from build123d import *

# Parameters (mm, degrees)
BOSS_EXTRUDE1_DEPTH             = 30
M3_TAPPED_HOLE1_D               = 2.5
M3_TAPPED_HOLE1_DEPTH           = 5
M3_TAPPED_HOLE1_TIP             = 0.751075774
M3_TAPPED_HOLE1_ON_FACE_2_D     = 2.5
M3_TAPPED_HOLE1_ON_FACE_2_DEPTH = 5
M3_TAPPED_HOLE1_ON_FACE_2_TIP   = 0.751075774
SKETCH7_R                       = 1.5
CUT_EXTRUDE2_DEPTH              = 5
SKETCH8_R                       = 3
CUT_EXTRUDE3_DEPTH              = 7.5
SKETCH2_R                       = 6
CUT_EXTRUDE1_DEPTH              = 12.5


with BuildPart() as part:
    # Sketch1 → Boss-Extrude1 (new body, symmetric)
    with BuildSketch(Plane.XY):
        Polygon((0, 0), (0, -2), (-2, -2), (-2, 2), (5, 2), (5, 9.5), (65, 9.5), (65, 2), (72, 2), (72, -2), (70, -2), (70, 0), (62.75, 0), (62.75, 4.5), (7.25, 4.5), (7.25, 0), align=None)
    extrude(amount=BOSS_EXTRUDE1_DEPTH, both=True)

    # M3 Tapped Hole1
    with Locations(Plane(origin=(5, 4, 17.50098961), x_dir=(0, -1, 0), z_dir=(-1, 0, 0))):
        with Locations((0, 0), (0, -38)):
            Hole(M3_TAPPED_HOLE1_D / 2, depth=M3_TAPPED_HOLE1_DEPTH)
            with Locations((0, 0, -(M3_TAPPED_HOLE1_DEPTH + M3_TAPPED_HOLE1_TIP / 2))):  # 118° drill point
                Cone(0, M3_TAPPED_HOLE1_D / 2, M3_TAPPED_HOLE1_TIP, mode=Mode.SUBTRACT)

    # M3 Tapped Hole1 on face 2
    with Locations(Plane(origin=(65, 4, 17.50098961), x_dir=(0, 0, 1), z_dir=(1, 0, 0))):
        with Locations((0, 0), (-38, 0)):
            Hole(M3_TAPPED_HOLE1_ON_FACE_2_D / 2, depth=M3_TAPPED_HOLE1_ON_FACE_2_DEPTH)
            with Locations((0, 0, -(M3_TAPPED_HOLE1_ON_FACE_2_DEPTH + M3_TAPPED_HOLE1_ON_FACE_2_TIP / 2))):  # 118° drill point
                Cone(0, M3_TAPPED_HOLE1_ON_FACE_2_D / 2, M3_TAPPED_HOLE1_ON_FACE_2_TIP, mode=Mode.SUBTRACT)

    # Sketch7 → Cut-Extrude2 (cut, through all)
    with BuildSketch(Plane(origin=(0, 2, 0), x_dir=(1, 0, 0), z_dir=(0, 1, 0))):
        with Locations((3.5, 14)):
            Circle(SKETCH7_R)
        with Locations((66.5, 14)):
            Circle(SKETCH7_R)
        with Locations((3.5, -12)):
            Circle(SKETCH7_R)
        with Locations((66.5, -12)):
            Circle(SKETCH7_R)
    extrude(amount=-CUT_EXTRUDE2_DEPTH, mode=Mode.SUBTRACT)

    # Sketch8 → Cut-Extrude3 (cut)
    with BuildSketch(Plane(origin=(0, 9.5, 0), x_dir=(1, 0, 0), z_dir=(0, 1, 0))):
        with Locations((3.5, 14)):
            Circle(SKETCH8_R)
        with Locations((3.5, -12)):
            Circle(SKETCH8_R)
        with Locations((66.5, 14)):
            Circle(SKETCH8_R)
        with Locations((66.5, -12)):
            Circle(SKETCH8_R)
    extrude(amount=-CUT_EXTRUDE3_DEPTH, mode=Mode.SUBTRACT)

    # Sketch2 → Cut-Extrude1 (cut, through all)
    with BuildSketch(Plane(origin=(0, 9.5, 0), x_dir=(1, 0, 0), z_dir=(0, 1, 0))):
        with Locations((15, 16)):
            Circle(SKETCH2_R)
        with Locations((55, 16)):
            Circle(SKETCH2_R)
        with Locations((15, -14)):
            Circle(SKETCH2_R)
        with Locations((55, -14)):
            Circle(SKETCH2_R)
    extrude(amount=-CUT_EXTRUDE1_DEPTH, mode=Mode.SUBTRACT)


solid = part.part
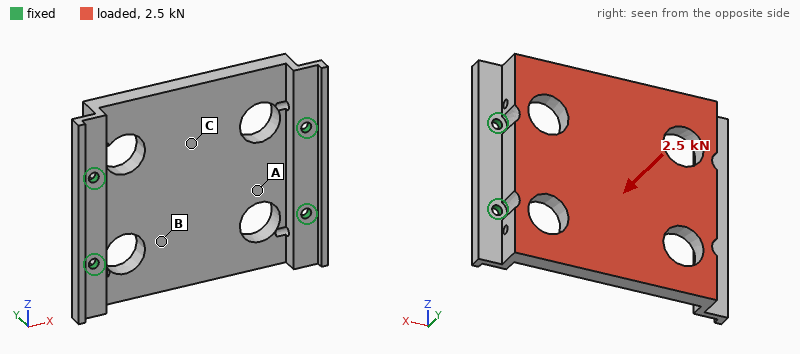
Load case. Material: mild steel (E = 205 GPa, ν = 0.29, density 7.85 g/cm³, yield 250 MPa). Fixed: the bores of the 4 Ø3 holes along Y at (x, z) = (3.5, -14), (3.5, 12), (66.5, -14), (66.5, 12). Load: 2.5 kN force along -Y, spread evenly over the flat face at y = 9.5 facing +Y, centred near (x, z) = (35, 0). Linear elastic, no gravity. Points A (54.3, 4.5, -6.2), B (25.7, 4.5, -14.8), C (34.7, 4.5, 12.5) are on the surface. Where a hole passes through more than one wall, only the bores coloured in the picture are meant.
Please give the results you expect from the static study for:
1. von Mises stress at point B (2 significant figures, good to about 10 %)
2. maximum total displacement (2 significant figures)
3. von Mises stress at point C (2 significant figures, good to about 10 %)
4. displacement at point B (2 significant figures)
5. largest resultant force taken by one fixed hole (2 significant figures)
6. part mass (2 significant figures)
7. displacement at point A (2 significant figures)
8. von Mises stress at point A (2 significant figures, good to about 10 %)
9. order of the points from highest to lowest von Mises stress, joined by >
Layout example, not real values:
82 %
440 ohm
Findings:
24 MPa
37 µm
37 MPa
25 µm
1.1 kN
150 g
13 µm
10 MPa
C > B > A
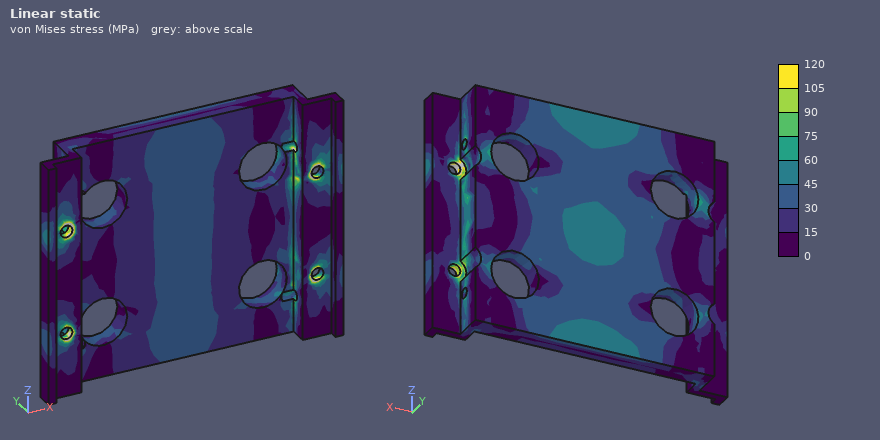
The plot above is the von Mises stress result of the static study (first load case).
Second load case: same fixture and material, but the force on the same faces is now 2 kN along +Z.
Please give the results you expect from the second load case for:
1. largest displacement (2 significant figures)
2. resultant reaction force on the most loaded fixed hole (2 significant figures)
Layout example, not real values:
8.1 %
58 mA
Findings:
12 µm
640 N
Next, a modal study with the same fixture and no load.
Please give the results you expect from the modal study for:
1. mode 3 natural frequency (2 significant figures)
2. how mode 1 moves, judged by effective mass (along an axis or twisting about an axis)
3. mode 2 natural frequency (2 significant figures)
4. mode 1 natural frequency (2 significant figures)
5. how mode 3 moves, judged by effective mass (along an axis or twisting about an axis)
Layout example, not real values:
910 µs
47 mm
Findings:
7400 Hz
along Y
4900 Hz
4500 Hz
along X
